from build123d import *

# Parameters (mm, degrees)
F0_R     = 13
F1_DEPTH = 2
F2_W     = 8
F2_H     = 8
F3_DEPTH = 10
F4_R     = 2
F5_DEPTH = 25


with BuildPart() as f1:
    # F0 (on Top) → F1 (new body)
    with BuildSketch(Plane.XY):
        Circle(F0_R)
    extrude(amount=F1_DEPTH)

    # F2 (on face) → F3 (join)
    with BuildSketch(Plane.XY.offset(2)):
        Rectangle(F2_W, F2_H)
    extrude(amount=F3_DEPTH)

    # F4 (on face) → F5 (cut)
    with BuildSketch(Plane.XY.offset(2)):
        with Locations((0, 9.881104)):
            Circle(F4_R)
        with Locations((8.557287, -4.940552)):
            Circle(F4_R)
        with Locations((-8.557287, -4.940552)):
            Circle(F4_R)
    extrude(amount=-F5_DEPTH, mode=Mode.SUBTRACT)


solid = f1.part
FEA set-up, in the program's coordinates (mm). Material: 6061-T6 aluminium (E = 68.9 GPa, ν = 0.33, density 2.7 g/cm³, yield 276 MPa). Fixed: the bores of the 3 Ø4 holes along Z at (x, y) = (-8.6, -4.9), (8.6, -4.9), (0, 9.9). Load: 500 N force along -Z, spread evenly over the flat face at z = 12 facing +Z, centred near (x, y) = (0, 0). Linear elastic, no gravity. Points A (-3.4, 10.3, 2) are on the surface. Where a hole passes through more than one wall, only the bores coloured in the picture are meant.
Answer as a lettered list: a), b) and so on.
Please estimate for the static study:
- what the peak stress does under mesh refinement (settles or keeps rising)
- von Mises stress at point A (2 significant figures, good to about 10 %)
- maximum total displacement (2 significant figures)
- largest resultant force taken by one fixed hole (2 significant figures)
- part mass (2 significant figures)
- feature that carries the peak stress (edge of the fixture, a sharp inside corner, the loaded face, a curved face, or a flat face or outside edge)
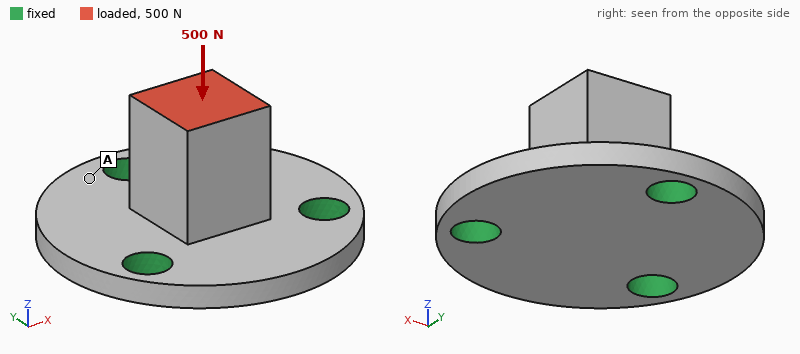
a) keeps rising
b) 10 MPa
c) 7.5 µm
d) 170 N
e) 4.4 g
f) edge of the fixture
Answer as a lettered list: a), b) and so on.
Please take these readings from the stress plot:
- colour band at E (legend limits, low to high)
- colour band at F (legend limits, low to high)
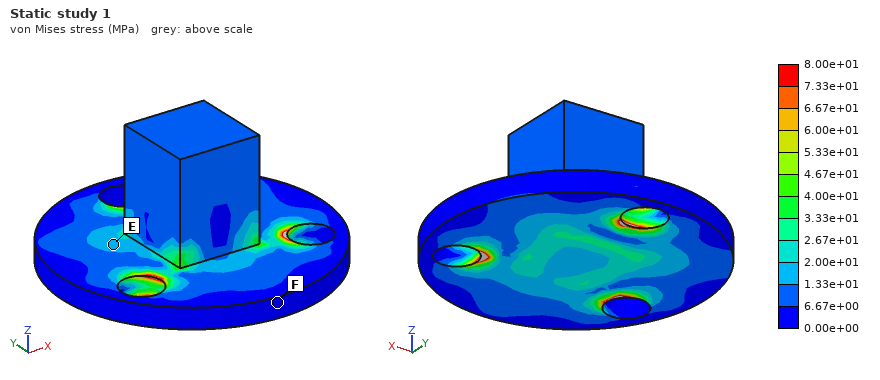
a) 1.33e+01 to 2.00e+01 MPa
b) 0.00e+00 to 6.67e+00 MPa
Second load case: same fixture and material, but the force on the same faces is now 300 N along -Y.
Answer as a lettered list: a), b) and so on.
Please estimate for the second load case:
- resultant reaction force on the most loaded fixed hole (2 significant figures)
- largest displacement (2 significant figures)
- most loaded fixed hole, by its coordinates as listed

a) 290 N
b) 26 µm
c) (0, 9.9)
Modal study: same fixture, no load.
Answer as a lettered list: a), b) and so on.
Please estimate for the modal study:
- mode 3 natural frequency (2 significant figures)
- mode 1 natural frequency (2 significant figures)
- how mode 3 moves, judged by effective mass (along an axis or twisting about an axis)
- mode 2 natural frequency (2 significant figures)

a) 27 kHz
b) 21 kHz
c) along Z
d) 21 kHz
